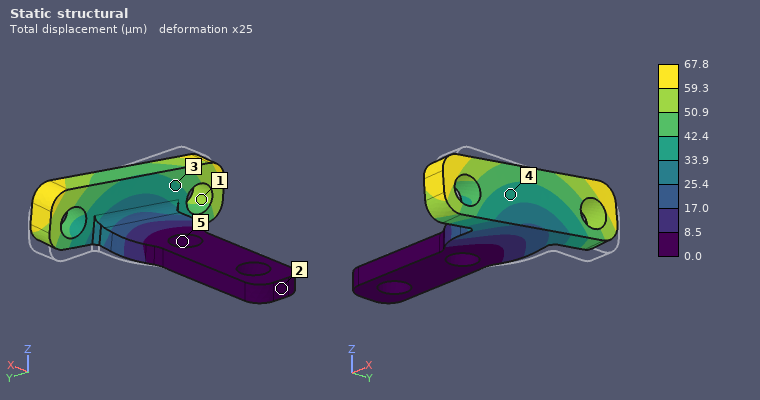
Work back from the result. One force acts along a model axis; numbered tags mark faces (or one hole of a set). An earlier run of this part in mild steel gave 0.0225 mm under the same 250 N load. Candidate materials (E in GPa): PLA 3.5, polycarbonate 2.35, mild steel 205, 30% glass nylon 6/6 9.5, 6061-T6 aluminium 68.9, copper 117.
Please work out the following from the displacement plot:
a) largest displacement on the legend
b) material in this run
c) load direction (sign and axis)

67.8 µm
6061-T6 aluminium
-Y
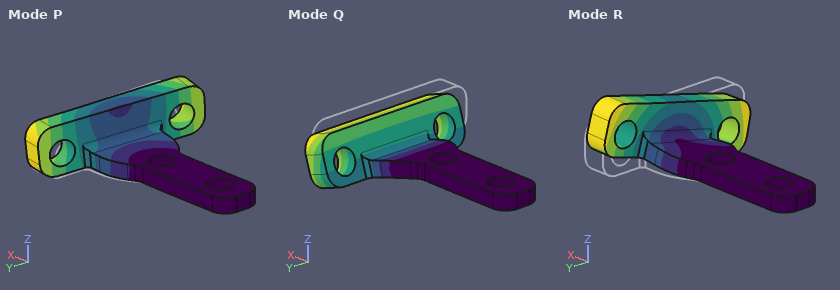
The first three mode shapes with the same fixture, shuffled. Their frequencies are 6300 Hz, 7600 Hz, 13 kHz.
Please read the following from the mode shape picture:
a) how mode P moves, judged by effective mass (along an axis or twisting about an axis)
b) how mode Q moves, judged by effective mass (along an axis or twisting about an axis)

along Y
along Z
